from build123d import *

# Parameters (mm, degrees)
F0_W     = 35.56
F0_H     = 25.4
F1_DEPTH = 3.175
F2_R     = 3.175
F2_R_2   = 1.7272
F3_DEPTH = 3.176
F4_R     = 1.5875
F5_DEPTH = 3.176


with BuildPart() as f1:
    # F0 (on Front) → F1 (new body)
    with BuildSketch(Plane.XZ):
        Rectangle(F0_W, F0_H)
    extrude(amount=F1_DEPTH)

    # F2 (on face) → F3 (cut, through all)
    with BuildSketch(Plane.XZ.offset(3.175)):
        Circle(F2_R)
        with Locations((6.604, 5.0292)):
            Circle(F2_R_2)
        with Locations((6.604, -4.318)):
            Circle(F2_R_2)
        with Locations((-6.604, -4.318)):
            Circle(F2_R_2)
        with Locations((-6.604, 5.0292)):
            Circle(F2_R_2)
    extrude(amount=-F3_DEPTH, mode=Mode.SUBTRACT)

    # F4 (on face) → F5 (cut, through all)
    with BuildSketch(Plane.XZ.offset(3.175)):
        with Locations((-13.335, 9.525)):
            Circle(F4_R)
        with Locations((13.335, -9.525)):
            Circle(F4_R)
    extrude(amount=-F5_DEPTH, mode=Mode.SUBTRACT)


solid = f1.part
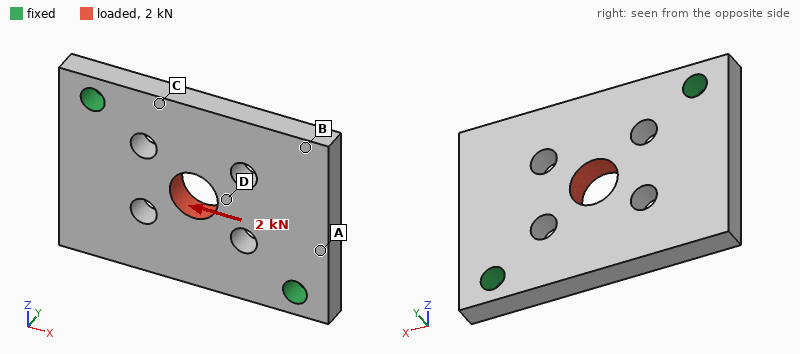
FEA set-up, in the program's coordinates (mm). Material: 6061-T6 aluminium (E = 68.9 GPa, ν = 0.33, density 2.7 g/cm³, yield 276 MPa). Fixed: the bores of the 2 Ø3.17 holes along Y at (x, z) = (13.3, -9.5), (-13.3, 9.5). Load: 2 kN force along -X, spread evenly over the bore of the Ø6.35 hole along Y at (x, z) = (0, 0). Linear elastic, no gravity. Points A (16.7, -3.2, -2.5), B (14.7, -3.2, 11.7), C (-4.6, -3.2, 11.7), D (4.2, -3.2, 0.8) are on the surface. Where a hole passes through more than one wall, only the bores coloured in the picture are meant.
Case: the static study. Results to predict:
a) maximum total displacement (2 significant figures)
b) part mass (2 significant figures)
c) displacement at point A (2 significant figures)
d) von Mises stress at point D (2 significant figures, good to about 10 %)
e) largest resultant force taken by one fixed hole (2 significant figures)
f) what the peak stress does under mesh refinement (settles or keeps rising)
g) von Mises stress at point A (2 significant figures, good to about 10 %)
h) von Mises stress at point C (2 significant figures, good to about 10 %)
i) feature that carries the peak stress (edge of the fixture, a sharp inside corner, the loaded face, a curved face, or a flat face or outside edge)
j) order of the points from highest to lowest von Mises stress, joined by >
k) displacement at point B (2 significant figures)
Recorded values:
11 µm
7.0 g
5.3 µm
37 MPa
1.0 kN
keeps rising
14 MPa
26 MPa
edge of the fixture
D > C > A > B
8.3 µm
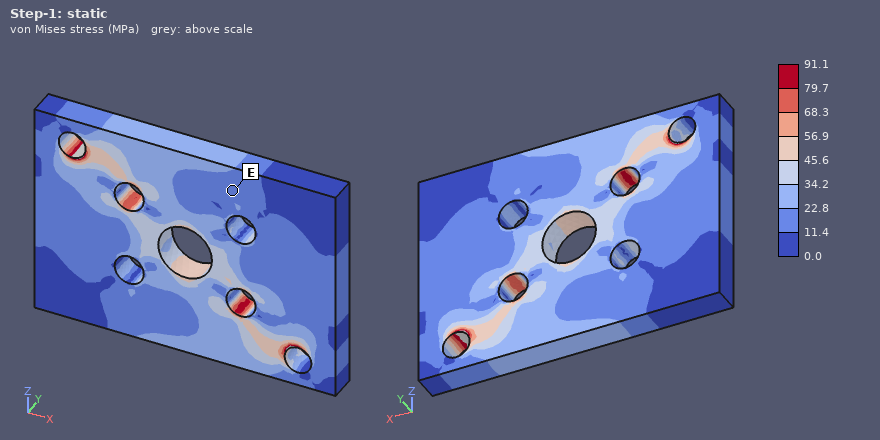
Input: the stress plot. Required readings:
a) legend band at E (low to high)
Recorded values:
11.4 to 22.8 MPa
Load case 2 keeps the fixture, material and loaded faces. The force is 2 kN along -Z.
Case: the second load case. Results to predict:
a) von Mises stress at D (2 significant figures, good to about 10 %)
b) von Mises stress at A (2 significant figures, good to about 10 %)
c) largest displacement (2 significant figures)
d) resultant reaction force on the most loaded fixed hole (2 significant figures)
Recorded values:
28 MPa
16 MPa
14 µm
1.0 kN
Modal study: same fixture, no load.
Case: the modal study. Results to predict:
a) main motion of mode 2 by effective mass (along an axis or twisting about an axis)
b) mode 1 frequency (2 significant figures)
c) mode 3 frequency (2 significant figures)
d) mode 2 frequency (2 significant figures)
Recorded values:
along Y
6500 Hz
17 kHz
8100 Hz
